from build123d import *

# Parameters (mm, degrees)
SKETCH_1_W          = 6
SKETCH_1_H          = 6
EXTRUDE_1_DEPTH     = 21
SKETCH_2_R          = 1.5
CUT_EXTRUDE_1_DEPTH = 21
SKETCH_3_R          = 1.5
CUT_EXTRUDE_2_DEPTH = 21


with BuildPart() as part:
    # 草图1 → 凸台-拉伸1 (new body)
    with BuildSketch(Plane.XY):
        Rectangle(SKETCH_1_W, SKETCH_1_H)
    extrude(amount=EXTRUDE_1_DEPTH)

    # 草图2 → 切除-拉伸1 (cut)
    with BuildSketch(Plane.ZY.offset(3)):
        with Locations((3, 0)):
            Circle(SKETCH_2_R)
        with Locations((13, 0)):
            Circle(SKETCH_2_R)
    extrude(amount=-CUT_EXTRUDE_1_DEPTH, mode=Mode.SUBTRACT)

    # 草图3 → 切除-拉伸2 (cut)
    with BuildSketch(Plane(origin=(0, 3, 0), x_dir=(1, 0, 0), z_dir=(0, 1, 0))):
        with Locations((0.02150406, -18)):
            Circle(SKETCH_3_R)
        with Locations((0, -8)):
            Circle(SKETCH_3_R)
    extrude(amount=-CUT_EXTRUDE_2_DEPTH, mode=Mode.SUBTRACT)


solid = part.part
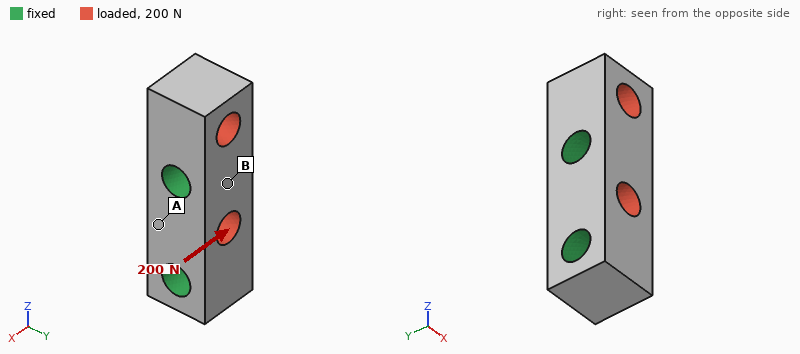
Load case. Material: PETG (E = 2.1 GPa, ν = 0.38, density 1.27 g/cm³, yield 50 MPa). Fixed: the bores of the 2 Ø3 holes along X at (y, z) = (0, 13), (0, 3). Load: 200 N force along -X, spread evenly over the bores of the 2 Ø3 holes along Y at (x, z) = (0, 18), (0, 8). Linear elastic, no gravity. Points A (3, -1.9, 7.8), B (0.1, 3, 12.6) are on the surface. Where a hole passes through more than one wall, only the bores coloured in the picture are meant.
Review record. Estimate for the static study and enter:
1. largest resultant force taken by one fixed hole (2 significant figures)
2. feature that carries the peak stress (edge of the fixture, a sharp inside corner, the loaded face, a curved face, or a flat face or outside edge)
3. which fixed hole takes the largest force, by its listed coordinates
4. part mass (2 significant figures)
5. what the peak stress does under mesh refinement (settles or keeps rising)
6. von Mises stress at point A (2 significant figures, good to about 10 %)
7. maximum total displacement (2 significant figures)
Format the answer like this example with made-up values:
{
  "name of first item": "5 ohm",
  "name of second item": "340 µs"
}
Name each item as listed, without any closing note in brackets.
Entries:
{
  "largest resultant force taken by one fixed hole": "150 N",
  "feature that carries the peak stress": "edge of the fixture",
  "which fixed hole takes the largest force, by its listed coordinates": "(0, 13)",
  "part mass": "0.74 g",
  "what the peak stress does under mesh refinement": "keeps rising",
  "von Mises stress at point A": "3.4 MPa",
  "maximum total displacement": "67 µm"
}
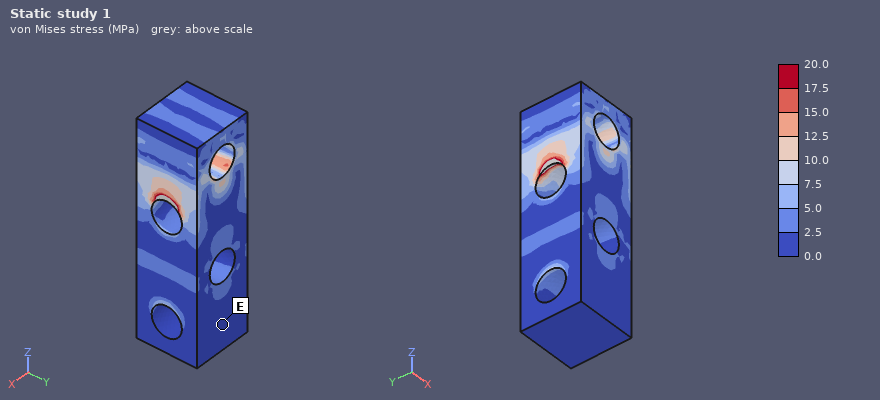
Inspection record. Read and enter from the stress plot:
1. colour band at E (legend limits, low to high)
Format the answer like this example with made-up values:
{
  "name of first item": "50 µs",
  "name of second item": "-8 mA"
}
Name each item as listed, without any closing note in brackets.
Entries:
{
  "colour band at E": "0.0 to 2.5 MPa"
}
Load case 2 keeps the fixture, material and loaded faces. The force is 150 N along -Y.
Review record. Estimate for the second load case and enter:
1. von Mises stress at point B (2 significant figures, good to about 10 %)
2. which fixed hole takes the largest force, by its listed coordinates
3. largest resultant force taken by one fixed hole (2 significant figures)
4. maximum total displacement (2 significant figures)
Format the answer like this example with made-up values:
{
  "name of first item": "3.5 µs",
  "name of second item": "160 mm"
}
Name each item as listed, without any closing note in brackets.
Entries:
{
  "von Mises stress at point B": "4.9 MPa",
  "which fixed hole takes the largest force, by its listed coordinates": "(0, 13)",
  "largest resultant force taken by one fixed hole": "120 N",
  "maximum total displacement": "53 µm"
}
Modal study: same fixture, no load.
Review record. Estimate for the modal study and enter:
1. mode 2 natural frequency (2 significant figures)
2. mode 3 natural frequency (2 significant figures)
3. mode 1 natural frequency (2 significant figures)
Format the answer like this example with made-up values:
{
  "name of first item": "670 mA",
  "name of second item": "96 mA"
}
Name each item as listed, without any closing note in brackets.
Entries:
{
  "mode 2 natural frequency": "15 kHz",
  "mode 3 natural frequency": "22 kHz",
  "mode 1 natural frequency": "14 kHz"
}
